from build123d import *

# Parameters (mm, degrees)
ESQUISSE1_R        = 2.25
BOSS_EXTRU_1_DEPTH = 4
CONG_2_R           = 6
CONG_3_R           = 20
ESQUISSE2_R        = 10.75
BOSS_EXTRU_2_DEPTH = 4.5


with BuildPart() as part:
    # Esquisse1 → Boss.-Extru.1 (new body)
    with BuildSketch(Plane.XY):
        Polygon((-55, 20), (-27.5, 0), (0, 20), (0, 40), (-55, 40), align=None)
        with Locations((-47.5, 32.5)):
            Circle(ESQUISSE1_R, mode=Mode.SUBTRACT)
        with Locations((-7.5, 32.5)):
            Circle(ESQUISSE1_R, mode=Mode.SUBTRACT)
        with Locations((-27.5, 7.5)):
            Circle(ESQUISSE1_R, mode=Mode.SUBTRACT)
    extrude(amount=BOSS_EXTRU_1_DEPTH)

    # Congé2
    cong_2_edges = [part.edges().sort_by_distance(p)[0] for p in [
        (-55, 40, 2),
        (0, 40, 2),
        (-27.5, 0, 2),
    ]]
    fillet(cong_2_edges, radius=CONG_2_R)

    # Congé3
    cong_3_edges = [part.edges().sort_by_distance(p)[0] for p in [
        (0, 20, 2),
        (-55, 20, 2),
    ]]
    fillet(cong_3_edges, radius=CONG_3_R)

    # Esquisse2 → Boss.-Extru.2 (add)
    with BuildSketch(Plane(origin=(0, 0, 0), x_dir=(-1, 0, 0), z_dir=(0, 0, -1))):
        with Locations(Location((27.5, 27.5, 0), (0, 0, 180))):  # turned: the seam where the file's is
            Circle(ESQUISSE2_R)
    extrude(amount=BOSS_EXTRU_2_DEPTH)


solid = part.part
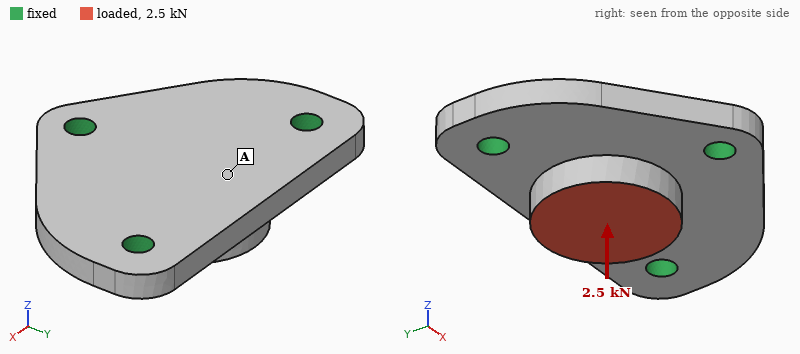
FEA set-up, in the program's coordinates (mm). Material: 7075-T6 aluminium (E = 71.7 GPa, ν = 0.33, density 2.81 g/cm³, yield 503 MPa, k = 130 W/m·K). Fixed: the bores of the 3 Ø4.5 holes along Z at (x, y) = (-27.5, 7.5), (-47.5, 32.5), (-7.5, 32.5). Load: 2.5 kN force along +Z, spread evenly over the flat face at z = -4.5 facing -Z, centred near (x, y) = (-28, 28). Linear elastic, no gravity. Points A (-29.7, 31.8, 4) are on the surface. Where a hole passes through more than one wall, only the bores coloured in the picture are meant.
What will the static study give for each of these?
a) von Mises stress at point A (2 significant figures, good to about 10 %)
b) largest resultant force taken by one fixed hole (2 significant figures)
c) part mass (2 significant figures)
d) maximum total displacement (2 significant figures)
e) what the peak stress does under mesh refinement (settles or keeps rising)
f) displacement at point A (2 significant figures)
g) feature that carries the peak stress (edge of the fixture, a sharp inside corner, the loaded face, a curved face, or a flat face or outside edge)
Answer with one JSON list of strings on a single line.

["30 MPa", "1.0 kN", "22 g", "41 µm", "keeps rising", "31 µm", "edge of the fixture"]
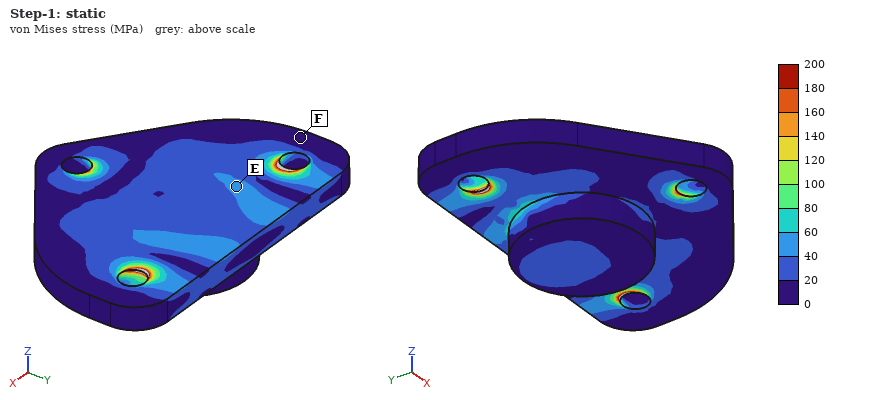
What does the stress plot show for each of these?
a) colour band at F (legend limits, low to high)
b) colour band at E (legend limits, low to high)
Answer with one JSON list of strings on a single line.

["0 to 20 MPa", "40 to 60 MPa"]
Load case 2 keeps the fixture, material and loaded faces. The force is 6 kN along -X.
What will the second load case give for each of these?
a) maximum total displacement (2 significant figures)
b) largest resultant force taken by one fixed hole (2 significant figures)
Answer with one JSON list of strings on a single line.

["32 µm", "2.7 kN"]
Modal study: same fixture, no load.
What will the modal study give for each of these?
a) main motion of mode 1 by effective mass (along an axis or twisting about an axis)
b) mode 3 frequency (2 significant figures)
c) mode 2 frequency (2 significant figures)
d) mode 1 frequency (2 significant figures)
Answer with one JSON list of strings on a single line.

["along Z", "18 kHz", "18 kHz", "14 kHz"]
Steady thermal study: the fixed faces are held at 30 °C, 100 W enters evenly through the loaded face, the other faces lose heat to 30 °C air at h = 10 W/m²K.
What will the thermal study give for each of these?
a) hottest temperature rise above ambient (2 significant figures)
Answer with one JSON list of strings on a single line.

["57 K"]
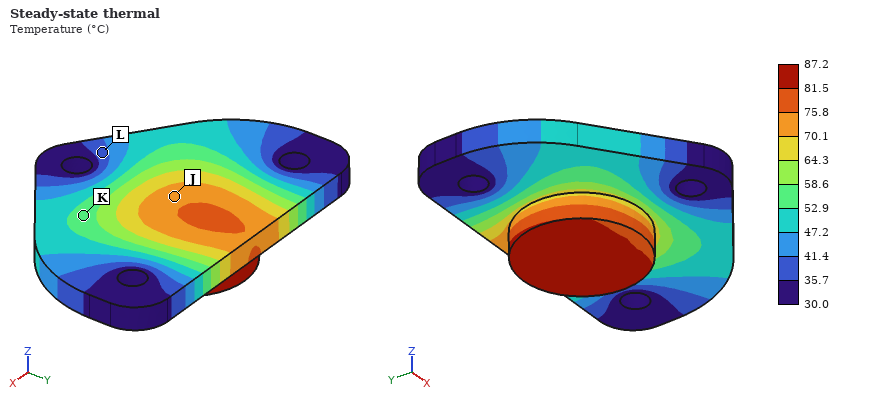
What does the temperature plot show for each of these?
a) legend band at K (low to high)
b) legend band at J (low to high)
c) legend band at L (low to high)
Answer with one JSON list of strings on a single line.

["52.9 to 58.6 °C", "70.1 to 75.8 °C", "35.7 to 41.4 °C"]
